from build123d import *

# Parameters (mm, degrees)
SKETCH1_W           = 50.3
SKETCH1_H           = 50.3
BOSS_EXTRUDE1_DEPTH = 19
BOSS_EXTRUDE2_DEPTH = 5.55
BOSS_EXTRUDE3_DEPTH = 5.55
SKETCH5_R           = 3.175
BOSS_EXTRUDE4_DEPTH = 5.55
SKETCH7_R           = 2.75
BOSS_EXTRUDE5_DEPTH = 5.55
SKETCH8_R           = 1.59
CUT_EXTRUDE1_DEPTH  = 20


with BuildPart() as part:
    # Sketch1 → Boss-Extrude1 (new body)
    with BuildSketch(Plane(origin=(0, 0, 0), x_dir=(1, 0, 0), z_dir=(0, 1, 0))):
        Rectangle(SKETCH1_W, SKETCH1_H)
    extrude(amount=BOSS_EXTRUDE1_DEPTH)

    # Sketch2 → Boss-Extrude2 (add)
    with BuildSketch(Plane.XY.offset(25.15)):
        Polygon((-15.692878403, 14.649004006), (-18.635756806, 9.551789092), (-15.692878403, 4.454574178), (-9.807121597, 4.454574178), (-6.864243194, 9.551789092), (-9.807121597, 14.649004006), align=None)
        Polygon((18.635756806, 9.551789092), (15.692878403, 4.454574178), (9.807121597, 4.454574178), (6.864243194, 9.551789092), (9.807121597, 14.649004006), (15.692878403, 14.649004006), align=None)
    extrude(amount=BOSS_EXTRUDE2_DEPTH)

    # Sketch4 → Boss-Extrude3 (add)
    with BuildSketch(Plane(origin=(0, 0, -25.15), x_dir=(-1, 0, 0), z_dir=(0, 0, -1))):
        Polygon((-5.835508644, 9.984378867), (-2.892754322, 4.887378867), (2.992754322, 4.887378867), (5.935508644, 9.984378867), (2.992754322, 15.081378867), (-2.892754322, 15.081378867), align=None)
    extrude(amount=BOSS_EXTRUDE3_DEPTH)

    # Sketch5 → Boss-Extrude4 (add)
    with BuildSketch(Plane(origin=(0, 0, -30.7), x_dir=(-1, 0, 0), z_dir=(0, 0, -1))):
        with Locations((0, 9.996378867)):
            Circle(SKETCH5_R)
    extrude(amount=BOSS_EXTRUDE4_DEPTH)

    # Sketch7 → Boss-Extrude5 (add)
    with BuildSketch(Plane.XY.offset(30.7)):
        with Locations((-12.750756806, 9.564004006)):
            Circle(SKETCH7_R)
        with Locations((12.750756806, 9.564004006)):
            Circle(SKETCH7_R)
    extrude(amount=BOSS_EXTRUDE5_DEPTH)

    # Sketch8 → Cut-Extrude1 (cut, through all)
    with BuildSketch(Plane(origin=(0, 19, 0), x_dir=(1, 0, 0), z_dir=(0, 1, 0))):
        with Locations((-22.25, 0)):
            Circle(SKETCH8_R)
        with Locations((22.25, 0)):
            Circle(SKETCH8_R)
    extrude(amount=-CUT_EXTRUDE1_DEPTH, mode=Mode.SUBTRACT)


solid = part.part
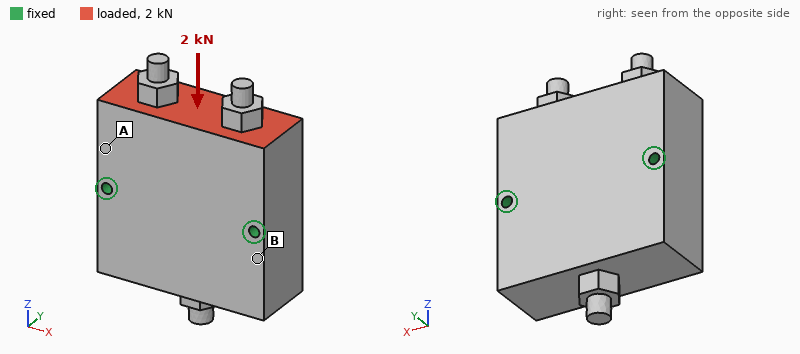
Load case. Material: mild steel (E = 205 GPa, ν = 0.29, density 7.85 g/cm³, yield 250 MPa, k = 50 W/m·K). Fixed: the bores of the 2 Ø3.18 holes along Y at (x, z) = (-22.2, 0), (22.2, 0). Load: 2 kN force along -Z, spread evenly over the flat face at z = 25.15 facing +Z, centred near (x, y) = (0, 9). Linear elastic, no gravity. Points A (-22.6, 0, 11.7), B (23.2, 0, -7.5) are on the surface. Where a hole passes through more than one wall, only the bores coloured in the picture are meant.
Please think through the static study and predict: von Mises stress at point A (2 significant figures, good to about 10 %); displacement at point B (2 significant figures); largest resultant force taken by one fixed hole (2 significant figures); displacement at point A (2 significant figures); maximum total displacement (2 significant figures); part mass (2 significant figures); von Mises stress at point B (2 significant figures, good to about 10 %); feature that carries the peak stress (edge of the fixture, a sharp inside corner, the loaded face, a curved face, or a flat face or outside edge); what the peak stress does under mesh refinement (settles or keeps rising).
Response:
3.0 MPa
0.074 µm
1.0 kN
0.21 µm
0.48 µm
390 g
1.4 MPa
edge of the fixture
keeps rising
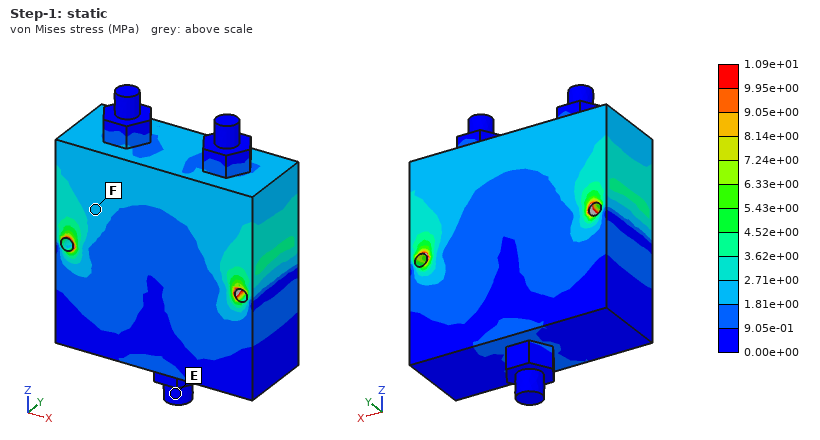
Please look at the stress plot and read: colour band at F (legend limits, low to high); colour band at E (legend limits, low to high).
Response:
1.81e+00 to 2.71e+00 MPa
0.00e+00 to 9.05e-01 MPa
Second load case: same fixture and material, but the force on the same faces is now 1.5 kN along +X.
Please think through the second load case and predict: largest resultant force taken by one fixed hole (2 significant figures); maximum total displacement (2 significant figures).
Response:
1.1 kN
1.1 µm
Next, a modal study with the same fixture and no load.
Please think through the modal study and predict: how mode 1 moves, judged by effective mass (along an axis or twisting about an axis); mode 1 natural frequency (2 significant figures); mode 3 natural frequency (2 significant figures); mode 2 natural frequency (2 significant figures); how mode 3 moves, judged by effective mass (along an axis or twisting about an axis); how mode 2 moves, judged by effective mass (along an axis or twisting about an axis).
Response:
twisting about X
10 kHz
20 kHz
13 kHz
along X
along Y
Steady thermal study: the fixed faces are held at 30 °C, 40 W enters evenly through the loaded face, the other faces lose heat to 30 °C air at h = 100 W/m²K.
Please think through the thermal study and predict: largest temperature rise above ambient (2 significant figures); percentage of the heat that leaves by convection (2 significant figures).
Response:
25 K
21 %
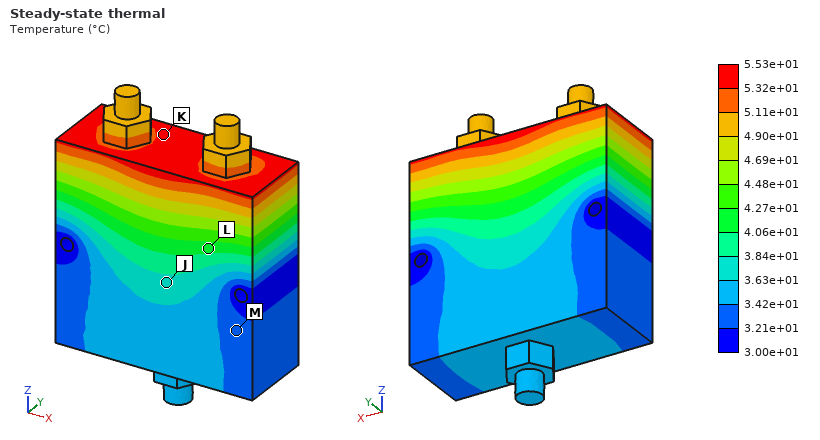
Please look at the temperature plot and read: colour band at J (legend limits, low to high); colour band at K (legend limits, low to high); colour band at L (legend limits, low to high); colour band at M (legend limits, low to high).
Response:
3.63e+01 to 3.84e+01 °C
5.32e+01 to 5.53e+01 °C
4.06e+01 to 4.27e+01 °C
3.21e+01 to 3.42e+01 °C
